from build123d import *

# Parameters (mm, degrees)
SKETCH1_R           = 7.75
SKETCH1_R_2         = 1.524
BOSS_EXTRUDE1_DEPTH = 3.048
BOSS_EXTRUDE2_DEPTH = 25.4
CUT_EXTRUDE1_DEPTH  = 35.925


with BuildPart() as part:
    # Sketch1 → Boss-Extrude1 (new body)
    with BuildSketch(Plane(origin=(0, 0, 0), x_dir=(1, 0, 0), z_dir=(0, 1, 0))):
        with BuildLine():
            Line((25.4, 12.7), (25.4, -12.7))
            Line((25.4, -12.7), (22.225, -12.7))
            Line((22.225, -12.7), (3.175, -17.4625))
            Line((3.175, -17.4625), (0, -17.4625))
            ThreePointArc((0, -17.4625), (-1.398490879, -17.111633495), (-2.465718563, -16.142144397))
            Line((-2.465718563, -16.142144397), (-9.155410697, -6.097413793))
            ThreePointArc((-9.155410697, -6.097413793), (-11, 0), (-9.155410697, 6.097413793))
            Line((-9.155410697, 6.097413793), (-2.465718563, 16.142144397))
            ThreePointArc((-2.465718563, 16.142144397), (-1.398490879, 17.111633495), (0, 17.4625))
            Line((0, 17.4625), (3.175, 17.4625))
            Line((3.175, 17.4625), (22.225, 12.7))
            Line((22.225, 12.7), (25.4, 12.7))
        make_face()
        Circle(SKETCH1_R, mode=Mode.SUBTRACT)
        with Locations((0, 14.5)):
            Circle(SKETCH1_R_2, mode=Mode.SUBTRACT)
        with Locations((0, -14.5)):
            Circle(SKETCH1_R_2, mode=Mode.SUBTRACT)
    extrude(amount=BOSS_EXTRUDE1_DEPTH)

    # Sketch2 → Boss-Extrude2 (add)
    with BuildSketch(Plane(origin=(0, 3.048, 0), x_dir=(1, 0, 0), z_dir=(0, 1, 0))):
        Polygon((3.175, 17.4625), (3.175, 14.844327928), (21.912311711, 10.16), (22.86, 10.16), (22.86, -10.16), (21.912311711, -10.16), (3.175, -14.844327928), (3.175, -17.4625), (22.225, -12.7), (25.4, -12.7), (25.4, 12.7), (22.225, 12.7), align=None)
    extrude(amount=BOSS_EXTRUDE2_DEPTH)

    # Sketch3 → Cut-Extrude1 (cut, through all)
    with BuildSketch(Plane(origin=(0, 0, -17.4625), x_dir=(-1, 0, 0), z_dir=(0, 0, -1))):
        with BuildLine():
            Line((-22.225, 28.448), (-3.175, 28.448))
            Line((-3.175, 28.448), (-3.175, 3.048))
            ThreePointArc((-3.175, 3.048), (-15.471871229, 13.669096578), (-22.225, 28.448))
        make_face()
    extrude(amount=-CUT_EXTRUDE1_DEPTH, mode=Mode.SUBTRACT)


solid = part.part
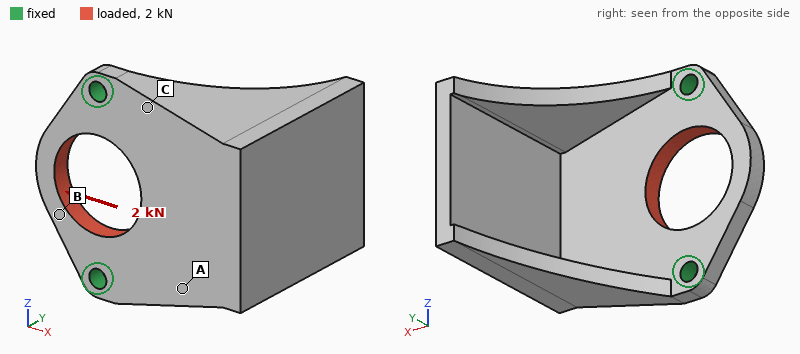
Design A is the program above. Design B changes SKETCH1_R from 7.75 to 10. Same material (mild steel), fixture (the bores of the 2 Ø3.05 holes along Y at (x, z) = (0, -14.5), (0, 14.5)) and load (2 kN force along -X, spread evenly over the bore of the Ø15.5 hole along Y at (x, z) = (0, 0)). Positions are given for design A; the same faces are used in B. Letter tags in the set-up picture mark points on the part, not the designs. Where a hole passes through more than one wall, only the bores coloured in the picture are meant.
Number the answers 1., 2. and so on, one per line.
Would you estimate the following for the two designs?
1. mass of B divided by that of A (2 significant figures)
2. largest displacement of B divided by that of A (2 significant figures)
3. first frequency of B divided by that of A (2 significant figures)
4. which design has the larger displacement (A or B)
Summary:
1. 0.92
2. 2.6
3. 0.94
4. B
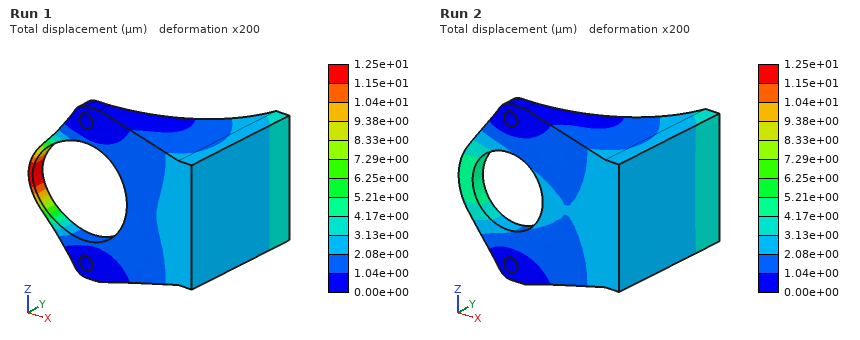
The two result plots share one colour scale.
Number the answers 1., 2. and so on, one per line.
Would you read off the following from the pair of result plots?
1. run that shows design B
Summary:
1. Run 1
